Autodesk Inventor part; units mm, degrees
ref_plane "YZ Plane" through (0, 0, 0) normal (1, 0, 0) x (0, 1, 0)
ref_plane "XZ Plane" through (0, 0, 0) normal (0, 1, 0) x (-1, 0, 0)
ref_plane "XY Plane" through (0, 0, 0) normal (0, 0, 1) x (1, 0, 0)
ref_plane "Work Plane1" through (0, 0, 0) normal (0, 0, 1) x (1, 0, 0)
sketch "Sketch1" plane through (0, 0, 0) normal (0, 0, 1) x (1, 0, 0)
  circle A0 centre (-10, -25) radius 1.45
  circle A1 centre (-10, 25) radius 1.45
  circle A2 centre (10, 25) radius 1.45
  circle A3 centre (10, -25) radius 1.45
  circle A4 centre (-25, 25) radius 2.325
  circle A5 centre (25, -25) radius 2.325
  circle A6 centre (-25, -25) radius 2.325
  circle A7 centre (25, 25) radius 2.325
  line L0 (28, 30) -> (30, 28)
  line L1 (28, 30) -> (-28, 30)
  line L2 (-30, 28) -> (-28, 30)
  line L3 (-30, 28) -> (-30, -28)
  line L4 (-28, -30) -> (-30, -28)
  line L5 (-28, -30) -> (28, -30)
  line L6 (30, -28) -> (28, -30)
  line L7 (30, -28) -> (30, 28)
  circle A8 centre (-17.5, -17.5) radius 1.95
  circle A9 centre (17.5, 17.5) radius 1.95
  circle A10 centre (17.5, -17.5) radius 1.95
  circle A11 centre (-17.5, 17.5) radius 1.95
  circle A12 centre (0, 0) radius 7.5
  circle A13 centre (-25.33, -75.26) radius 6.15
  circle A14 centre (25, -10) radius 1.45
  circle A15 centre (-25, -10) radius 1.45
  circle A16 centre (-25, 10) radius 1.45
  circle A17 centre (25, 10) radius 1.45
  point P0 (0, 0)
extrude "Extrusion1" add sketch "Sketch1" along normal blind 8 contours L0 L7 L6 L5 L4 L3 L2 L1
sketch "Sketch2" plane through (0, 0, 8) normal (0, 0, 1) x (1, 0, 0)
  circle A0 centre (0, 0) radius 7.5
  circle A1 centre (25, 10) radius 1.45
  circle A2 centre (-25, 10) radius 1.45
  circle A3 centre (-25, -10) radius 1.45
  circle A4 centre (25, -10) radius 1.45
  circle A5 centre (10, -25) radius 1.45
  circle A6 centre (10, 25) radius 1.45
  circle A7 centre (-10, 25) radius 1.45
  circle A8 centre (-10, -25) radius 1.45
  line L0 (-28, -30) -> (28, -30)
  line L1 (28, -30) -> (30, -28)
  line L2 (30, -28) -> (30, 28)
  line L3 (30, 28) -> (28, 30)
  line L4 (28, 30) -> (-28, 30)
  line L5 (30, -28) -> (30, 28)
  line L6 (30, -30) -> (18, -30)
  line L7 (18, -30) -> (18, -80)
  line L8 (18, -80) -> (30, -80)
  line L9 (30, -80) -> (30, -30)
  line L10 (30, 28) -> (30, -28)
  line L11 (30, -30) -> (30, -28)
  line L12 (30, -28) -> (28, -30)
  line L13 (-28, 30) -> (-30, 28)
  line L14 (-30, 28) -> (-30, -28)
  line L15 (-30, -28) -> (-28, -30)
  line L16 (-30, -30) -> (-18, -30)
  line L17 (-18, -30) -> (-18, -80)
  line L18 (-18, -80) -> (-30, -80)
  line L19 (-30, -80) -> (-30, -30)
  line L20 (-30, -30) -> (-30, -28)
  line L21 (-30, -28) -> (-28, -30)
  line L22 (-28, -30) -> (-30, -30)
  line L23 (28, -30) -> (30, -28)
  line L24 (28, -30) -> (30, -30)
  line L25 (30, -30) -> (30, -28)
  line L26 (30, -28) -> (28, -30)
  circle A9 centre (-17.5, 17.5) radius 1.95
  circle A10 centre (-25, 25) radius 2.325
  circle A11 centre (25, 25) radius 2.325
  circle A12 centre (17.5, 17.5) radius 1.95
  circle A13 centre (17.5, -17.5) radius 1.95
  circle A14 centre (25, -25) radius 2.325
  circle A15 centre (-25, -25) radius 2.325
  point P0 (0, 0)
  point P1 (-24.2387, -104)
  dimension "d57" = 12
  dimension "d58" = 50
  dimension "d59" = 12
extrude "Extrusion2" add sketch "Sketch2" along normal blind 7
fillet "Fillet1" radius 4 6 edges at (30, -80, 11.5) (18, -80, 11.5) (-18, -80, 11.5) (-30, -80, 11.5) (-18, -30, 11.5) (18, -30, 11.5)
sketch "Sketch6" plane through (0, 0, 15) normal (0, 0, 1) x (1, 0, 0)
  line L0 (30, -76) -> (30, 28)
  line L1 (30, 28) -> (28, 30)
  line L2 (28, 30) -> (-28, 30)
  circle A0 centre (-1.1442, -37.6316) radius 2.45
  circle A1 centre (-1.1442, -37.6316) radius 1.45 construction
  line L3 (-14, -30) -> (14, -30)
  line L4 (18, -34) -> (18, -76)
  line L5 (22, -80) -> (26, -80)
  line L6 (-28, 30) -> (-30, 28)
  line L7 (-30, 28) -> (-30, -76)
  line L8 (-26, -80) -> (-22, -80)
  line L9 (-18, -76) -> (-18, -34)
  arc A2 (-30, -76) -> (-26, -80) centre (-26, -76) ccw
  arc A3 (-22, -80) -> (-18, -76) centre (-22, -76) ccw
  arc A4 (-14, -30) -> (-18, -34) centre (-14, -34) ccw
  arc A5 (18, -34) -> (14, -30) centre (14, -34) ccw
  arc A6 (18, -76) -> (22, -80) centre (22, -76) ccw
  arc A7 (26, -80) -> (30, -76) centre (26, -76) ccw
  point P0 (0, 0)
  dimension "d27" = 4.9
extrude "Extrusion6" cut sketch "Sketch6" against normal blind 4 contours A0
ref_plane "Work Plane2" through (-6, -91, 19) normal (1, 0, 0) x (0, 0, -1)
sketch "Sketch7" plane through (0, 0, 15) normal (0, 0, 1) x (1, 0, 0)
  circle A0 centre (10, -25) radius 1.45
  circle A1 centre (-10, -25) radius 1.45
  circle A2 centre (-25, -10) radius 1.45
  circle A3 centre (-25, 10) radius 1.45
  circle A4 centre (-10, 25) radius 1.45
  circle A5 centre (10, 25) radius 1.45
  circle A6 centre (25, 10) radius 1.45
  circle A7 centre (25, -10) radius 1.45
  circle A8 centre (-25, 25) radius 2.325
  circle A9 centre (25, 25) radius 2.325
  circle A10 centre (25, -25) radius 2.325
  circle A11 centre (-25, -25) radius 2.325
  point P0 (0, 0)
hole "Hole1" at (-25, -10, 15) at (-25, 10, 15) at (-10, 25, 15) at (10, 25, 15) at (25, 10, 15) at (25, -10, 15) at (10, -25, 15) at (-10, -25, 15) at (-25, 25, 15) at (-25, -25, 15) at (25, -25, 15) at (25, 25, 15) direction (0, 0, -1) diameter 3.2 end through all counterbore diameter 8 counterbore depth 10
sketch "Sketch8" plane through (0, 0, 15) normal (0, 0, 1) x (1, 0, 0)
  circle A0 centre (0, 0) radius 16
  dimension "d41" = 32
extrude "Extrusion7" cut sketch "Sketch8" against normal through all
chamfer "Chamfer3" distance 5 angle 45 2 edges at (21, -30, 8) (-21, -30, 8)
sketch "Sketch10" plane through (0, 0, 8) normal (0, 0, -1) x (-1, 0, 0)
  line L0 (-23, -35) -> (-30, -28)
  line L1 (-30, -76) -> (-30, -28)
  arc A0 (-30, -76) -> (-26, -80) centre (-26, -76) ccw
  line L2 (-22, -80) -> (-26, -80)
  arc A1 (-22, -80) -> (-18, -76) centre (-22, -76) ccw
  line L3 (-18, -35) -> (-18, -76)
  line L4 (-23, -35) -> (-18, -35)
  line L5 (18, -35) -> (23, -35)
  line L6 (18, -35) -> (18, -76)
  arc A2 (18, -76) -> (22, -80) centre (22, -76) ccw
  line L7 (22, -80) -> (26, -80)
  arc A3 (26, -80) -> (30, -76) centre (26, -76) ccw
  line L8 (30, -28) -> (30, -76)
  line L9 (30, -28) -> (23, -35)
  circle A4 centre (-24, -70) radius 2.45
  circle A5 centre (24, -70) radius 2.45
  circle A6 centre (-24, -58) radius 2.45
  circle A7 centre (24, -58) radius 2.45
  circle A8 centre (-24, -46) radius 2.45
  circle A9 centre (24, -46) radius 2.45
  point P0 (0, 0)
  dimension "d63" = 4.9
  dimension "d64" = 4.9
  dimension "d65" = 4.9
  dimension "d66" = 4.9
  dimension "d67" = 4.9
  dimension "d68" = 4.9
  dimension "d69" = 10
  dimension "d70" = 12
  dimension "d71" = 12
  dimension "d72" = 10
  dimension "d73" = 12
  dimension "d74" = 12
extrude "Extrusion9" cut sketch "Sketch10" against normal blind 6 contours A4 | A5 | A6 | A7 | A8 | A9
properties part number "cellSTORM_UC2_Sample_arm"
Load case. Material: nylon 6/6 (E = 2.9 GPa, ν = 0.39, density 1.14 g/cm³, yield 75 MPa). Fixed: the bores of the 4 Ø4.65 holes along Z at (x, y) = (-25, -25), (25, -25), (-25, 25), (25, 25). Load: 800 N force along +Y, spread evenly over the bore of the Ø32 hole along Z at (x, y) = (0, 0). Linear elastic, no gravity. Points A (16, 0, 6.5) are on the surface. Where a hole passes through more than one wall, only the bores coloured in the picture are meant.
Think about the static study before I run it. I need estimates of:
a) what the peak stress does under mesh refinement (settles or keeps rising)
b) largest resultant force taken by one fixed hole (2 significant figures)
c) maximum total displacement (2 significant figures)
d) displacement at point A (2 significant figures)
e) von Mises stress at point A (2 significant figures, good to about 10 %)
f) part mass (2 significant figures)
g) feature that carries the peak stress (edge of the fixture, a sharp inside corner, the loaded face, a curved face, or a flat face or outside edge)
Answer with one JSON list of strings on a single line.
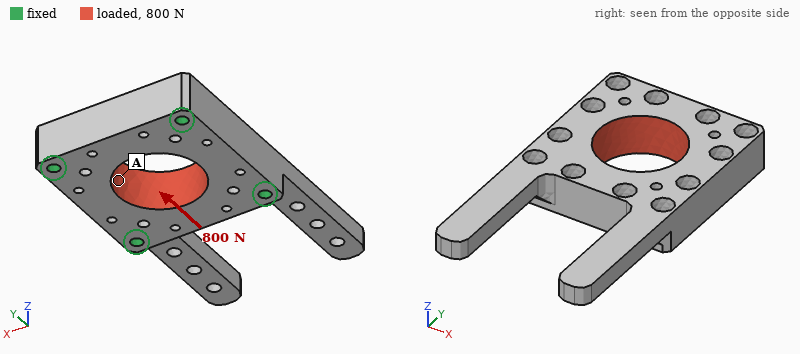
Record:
["keeps rising", "210 N", "56 µm", "15 µm", "1.3 MPa", "48 g", "edge of the fixture"]
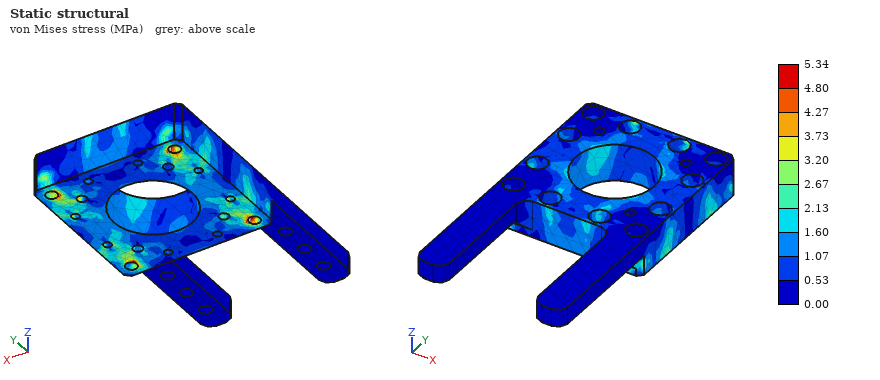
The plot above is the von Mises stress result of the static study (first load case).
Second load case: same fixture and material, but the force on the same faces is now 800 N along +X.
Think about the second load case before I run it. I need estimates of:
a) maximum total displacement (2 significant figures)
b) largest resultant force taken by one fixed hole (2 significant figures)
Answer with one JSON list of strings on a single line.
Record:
["30 µm", "210 N"]
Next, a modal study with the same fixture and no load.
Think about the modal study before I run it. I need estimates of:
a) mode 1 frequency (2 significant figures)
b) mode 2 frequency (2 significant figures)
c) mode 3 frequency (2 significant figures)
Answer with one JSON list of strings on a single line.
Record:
["670 Hz", "680 Hz", "990 Hz"]
